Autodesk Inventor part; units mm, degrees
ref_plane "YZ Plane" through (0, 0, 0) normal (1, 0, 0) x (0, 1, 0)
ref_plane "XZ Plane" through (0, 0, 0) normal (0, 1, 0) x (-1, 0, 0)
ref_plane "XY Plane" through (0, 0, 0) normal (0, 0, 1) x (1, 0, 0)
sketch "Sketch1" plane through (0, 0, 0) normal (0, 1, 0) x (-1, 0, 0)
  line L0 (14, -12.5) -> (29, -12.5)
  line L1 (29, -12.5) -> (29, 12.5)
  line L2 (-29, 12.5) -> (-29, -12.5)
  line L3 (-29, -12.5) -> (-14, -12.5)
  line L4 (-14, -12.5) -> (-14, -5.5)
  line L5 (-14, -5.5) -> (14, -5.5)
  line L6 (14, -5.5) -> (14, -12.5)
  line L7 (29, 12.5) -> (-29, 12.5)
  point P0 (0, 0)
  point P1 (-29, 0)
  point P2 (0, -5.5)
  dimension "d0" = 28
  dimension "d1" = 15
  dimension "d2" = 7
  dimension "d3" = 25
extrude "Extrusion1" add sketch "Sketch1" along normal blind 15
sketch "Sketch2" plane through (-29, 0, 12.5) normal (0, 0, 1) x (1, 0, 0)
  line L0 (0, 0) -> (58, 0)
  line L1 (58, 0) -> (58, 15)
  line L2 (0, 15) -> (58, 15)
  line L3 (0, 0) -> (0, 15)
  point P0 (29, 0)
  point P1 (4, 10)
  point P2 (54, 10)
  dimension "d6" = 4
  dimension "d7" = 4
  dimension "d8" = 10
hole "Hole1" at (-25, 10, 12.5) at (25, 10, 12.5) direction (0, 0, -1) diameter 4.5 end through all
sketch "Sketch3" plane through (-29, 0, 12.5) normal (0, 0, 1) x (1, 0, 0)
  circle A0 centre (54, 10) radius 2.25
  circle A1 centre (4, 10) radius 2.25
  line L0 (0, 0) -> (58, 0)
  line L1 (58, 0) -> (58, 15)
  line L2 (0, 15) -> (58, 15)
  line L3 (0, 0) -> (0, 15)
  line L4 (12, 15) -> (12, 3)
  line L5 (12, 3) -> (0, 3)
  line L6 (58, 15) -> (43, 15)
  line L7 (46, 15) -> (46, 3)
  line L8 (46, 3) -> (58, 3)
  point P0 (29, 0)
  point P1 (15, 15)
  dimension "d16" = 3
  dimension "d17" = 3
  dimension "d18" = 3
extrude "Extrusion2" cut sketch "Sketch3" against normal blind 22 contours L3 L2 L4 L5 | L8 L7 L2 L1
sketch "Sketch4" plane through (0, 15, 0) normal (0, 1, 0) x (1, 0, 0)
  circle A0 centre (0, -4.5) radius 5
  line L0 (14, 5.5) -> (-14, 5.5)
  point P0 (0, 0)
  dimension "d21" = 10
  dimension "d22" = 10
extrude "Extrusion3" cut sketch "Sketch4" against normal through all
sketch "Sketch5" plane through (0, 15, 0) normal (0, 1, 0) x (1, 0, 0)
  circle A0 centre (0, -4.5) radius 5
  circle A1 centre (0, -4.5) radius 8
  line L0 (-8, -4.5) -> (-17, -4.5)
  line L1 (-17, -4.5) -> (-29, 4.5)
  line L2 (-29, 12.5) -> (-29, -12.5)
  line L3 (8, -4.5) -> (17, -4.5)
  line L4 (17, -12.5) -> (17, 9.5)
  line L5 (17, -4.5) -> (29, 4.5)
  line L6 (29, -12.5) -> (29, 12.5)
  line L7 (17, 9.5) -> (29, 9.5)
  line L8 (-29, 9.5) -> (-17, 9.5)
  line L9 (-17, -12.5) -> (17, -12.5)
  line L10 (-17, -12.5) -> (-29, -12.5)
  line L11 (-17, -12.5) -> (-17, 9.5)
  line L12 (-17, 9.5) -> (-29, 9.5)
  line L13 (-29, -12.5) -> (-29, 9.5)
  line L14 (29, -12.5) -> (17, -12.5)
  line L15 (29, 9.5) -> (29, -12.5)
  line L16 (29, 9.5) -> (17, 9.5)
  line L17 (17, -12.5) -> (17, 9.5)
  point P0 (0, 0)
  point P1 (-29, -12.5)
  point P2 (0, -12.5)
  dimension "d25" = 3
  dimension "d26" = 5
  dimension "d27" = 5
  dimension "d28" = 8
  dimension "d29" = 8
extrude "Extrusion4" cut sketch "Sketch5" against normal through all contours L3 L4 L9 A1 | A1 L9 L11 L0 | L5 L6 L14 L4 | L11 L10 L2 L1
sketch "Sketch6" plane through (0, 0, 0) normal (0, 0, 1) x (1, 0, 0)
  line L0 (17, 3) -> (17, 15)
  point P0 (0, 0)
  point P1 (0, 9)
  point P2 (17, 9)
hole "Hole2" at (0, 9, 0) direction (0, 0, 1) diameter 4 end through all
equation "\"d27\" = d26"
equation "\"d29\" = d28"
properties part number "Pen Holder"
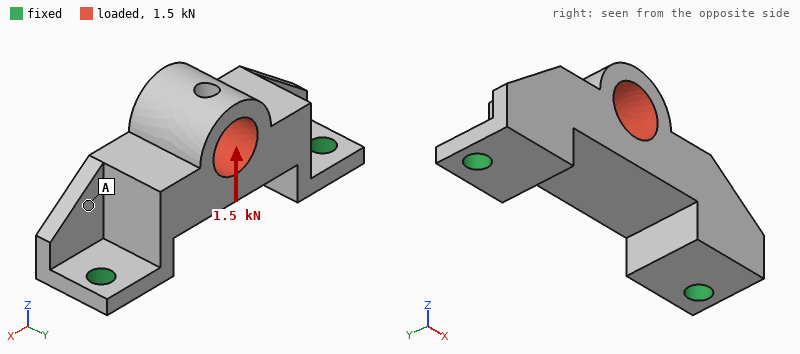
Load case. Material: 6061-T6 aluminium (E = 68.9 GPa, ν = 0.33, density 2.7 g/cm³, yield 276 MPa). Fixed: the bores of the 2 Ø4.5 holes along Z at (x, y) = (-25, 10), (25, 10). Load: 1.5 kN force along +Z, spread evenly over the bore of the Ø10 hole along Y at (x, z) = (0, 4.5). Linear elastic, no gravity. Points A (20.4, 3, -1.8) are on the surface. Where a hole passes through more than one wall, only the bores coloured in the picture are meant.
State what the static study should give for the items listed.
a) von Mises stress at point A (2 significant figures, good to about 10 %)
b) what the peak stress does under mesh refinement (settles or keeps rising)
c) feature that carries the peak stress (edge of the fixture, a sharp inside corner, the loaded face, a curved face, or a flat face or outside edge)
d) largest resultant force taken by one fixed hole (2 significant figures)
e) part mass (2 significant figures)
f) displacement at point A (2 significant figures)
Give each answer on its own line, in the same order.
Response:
17 MPa
keeps rising
edge of the fixture
1.0 kN
21 g
24 µm
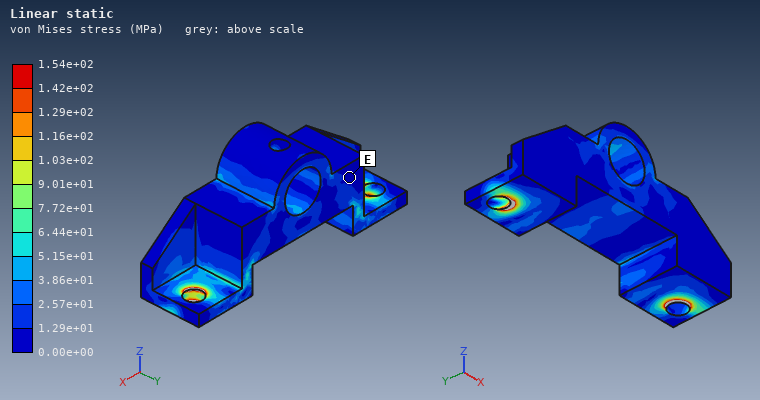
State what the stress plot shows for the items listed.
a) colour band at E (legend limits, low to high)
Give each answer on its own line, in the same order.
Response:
0.00e+00 to 1.29e+01 MPa
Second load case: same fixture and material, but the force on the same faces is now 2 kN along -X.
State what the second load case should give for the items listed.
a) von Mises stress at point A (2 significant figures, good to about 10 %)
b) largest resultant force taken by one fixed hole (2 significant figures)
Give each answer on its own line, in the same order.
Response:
18 MPa
1.2 kN
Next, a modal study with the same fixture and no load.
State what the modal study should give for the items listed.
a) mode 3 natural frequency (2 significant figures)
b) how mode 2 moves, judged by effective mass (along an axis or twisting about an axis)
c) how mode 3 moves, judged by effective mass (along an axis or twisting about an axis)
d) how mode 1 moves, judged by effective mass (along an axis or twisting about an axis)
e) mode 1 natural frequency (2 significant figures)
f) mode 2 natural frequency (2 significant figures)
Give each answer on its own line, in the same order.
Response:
11 kHz
along Z
along X
along Y
3300 Hz
9300 Hz
